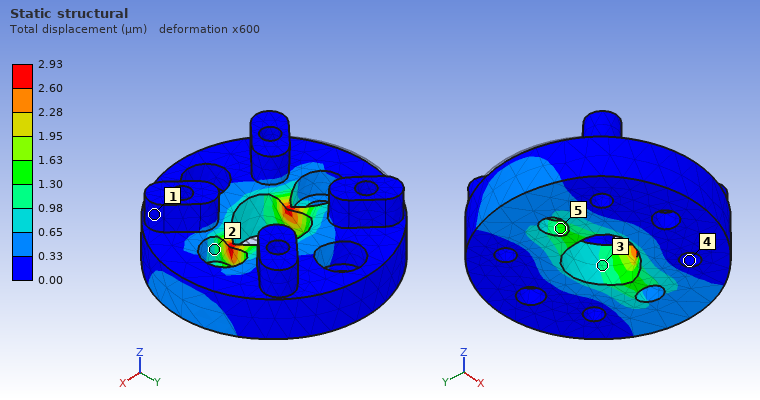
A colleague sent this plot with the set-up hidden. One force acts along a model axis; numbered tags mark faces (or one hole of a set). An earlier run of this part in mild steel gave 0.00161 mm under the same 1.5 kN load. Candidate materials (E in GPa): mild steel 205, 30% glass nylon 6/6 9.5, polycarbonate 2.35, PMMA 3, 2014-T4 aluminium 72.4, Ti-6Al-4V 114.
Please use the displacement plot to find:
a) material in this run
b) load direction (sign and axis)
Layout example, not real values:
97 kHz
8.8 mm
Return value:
Ti-6Al-4V
+X
